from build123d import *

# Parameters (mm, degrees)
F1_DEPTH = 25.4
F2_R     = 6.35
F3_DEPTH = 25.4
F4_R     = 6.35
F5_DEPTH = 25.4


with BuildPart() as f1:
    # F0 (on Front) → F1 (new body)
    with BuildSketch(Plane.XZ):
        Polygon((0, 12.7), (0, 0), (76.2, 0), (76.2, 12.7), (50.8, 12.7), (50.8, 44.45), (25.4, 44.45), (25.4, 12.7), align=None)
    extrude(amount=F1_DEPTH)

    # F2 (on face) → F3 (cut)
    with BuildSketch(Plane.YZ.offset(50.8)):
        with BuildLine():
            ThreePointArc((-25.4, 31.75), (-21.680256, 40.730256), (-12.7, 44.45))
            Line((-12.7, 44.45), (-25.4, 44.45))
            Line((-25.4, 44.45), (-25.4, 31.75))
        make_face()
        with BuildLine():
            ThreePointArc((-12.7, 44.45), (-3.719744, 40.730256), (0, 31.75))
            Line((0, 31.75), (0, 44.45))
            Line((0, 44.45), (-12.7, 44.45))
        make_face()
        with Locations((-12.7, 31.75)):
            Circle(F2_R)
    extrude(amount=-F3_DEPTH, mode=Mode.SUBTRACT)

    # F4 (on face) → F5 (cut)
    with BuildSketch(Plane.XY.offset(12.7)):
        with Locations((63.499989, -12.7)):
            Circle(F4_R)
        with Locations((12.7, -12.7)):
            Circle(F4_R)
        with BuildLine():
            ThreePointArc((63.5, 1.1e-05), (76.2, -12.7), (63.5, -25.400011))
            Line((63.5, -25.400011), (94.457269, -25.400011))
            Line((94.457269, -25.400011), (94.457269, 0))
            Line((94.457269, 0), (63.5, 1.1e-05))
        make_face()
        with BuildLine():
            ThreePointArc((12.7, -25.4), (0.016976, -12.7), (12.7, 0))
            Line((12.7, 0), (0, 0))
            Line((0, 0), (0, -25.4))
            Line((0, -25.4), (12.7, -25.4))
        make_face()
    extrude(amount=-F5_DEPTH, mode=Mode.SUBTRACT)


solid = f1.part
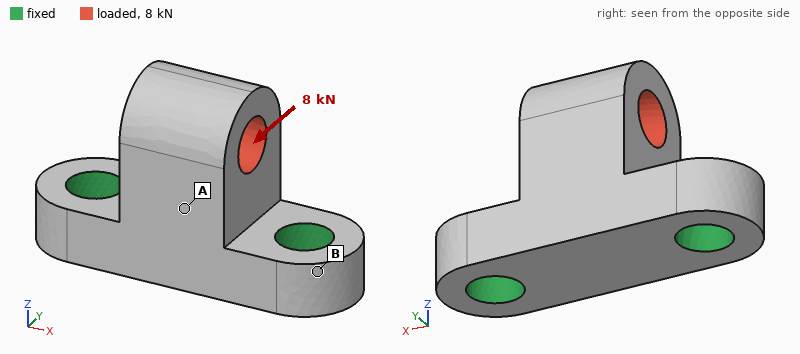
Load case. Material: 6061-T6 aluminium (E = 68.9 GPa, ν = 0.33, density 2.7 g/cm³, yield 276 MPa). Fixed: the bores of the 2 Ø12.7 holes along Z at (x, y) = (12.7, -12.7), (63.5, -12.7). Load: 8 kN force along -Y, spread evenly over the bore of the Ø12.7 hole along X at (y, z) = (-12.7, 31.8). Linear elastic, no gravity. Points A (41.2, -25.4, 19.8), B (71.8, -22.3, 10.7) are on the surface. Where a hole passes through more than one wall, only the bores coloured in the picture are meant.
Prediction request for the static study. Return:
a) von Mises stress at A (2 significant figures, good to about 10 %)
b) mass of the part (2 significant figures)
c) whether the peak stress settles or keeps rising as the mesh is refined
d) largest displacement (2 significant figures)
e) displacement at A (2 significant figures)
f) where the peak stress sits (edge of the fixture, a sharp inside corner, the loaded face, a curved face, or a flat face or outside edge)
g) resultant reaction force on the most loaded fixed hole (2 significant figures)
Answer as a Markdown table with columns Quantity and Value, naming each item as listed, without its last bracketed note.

| Quantity | Value |
|---|---|
| von Mises stress at A | 40 MPa |
| mass of the part | 95 g |
| whether the peak stress settles or keeps rising as the mesh is refined | keeps rising |
| largest displacement | 0.18 mm |
| displacement at A | 0.078 mm |
| where the peak stress sits | edge of the fixture |
| resultant reaction force on the most loaded fixed hole | 4.0 kN |
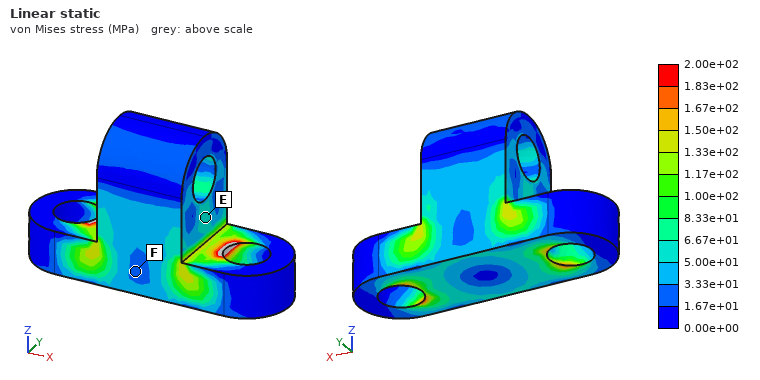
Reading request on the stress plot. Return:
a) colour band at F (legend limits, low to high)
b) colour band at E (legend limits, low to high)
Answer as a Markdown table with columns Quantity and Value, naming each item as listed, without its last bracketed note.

| Quantity | Value |
|---|---|
| colour band at F | 1.67e+01 to 3.33e+01 MPa |
| colour band at E | 5.00e+01 to 6.67e+01 MPa |
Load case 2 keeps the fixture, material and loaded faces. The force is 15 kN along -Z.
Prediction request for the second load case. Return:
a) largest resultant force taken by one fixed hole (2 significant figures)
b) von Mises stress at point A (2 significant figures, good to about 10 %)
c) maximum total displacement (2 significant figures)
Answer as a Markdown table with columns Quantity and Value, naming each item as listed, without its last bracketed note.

| Quantity | Value |
|---|---|
| largest resultant force taken by one fixed hole | 7.8 kN |
| von Mises stress at point A | 23 MPa |
| maximum total displacement | 34 µm |
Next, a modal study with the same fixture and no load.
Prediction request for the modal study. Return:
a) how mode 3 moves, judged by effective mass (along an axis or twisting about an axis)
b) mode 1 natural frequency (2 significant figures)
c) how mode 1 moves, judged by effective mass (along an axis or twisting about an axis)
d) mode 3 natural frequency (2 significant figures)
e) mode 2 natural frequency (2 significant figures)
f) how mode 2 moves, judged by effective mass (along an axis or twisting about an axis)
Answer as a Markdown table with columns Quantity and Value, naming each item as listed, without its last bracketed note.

| Quantity | Value |
|---|---|
| how mode 3 moves, judged by effective mass | along Z |
| mode 1 natural frequency | 6900 Hz |
| how mode 1 moves, judged by effective mass | along Y |
| mode 3 natural frequency | 17 kHz |
| mode 2 natural frequency | 12 kHz |
| how mode 2 moves, judged by effective mass | along X |
